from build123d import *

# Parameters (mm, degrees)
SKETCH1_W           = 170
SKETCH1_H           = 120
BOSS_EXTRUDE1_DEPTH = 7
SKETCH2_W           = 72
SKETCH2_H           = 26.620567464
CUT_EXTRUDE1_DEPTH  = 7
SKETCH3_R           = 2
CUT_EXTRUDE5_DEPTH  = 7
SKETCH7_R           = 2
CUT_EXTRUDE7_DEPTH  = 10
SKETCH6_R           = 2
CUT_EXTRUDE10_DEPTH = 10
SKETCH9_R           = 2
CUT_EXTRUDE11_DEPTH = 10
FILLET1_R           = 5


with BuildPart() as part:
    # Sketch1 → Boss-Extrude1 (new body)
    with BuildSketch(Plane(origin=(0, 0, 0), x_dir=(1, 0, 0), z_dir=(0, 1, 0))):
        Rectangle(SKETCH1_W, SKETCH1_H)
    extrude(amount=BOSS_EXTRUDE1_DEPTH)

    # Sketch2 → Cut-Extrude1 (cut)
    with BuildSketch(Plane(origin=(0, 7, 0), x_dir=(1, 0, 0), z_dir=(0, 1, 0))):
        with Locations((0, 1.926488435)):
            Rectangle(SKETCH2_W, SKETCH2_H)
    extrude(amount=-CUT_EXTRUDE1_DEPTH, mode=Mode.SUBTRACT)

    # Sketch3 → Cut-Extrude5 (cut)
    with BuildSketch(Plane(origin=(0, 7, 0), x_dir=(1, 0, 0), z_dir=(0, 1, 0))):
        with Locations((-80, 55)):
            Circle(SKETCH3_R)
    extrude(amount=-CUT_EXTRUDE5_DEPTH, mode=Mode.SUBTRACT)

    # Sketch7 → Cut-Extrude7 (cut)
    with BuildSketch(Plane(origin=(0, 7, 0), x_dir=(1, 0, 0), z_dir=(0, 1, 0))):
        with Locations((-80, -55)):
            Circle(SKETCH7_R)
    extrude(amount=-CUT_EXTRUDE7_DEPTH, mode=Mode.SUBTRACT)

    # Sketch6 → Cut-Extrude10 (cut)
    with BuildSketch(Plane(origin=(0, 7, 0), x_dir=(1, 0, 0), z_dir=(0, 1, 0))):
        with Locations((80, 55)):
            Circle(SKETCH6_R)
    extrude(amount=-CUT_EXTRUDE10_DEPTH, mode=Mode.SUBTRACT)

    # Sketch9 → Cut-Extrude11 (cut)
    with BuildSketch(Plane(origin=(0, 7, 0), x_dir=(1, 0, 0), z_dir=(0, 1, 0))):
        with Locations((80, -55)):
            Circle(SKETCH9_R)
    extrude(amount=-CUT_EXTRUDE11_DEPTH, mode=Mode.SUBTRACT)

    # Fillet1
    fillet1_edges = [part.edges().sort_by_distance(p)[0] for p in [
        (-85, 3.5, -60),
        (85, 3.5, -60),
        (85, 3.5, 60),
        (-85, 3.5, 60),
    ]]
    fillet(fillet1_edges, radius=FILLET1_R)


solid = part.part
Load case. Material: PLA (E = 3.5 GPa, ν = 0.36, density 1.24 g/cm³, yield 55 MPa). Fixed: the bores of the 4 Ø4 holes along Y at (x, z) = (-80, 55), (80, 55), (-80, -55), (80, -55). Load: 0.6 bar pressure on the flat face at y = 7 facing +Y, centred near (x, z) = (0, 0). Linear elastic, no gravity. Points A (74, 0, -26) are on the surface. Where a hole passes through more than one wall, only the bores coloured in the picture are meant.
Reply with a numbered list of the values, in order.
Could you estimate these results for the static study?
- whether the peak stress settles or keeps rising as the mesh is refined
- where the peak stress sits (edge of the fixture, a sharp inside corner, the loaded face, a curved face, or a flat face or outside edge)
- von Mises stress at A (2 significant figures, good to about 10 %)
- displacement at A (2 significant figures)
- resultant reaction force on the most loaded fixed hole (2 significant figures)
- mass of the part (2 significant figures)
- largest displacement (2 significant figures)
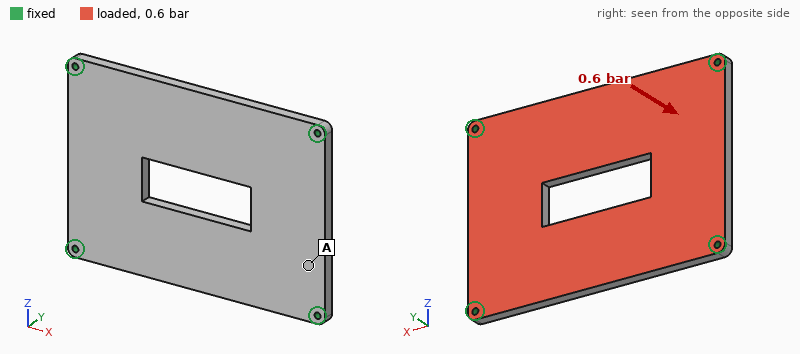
1. keeps rising
2. edge of the fixture
3. 4.4 MPa
4. 0.49 mm
5. 280 N
6. 160 g
7. 2.5 mm
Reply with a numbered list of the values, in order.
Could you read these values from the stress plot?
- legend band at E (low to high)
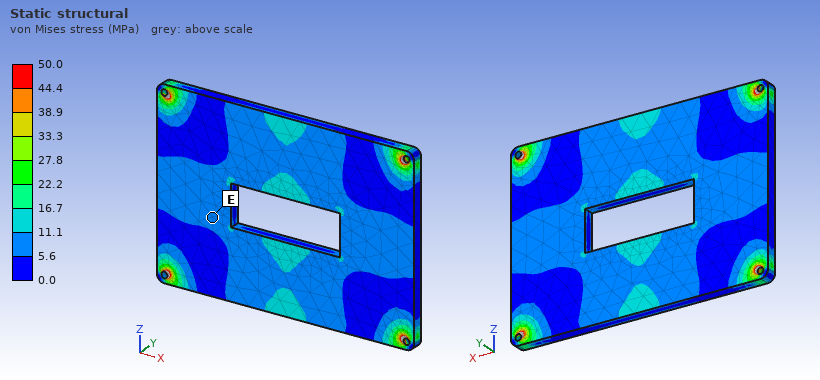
1. 5.6 to 11.1 MPa
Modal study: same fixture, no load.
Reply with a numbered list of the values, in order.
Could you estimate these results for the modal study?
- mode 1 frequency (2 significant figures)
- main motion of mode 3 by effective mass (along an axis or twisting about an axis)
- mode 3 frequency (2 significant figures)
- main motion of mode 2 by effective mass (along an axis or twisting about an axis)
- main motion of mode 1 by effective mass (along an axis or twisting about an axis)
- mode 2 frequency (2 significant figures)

1. 330 Hz
2. twisting about Z
3. 780 Hz
4. twisting about X
5. along Y
6. 530 Hz
